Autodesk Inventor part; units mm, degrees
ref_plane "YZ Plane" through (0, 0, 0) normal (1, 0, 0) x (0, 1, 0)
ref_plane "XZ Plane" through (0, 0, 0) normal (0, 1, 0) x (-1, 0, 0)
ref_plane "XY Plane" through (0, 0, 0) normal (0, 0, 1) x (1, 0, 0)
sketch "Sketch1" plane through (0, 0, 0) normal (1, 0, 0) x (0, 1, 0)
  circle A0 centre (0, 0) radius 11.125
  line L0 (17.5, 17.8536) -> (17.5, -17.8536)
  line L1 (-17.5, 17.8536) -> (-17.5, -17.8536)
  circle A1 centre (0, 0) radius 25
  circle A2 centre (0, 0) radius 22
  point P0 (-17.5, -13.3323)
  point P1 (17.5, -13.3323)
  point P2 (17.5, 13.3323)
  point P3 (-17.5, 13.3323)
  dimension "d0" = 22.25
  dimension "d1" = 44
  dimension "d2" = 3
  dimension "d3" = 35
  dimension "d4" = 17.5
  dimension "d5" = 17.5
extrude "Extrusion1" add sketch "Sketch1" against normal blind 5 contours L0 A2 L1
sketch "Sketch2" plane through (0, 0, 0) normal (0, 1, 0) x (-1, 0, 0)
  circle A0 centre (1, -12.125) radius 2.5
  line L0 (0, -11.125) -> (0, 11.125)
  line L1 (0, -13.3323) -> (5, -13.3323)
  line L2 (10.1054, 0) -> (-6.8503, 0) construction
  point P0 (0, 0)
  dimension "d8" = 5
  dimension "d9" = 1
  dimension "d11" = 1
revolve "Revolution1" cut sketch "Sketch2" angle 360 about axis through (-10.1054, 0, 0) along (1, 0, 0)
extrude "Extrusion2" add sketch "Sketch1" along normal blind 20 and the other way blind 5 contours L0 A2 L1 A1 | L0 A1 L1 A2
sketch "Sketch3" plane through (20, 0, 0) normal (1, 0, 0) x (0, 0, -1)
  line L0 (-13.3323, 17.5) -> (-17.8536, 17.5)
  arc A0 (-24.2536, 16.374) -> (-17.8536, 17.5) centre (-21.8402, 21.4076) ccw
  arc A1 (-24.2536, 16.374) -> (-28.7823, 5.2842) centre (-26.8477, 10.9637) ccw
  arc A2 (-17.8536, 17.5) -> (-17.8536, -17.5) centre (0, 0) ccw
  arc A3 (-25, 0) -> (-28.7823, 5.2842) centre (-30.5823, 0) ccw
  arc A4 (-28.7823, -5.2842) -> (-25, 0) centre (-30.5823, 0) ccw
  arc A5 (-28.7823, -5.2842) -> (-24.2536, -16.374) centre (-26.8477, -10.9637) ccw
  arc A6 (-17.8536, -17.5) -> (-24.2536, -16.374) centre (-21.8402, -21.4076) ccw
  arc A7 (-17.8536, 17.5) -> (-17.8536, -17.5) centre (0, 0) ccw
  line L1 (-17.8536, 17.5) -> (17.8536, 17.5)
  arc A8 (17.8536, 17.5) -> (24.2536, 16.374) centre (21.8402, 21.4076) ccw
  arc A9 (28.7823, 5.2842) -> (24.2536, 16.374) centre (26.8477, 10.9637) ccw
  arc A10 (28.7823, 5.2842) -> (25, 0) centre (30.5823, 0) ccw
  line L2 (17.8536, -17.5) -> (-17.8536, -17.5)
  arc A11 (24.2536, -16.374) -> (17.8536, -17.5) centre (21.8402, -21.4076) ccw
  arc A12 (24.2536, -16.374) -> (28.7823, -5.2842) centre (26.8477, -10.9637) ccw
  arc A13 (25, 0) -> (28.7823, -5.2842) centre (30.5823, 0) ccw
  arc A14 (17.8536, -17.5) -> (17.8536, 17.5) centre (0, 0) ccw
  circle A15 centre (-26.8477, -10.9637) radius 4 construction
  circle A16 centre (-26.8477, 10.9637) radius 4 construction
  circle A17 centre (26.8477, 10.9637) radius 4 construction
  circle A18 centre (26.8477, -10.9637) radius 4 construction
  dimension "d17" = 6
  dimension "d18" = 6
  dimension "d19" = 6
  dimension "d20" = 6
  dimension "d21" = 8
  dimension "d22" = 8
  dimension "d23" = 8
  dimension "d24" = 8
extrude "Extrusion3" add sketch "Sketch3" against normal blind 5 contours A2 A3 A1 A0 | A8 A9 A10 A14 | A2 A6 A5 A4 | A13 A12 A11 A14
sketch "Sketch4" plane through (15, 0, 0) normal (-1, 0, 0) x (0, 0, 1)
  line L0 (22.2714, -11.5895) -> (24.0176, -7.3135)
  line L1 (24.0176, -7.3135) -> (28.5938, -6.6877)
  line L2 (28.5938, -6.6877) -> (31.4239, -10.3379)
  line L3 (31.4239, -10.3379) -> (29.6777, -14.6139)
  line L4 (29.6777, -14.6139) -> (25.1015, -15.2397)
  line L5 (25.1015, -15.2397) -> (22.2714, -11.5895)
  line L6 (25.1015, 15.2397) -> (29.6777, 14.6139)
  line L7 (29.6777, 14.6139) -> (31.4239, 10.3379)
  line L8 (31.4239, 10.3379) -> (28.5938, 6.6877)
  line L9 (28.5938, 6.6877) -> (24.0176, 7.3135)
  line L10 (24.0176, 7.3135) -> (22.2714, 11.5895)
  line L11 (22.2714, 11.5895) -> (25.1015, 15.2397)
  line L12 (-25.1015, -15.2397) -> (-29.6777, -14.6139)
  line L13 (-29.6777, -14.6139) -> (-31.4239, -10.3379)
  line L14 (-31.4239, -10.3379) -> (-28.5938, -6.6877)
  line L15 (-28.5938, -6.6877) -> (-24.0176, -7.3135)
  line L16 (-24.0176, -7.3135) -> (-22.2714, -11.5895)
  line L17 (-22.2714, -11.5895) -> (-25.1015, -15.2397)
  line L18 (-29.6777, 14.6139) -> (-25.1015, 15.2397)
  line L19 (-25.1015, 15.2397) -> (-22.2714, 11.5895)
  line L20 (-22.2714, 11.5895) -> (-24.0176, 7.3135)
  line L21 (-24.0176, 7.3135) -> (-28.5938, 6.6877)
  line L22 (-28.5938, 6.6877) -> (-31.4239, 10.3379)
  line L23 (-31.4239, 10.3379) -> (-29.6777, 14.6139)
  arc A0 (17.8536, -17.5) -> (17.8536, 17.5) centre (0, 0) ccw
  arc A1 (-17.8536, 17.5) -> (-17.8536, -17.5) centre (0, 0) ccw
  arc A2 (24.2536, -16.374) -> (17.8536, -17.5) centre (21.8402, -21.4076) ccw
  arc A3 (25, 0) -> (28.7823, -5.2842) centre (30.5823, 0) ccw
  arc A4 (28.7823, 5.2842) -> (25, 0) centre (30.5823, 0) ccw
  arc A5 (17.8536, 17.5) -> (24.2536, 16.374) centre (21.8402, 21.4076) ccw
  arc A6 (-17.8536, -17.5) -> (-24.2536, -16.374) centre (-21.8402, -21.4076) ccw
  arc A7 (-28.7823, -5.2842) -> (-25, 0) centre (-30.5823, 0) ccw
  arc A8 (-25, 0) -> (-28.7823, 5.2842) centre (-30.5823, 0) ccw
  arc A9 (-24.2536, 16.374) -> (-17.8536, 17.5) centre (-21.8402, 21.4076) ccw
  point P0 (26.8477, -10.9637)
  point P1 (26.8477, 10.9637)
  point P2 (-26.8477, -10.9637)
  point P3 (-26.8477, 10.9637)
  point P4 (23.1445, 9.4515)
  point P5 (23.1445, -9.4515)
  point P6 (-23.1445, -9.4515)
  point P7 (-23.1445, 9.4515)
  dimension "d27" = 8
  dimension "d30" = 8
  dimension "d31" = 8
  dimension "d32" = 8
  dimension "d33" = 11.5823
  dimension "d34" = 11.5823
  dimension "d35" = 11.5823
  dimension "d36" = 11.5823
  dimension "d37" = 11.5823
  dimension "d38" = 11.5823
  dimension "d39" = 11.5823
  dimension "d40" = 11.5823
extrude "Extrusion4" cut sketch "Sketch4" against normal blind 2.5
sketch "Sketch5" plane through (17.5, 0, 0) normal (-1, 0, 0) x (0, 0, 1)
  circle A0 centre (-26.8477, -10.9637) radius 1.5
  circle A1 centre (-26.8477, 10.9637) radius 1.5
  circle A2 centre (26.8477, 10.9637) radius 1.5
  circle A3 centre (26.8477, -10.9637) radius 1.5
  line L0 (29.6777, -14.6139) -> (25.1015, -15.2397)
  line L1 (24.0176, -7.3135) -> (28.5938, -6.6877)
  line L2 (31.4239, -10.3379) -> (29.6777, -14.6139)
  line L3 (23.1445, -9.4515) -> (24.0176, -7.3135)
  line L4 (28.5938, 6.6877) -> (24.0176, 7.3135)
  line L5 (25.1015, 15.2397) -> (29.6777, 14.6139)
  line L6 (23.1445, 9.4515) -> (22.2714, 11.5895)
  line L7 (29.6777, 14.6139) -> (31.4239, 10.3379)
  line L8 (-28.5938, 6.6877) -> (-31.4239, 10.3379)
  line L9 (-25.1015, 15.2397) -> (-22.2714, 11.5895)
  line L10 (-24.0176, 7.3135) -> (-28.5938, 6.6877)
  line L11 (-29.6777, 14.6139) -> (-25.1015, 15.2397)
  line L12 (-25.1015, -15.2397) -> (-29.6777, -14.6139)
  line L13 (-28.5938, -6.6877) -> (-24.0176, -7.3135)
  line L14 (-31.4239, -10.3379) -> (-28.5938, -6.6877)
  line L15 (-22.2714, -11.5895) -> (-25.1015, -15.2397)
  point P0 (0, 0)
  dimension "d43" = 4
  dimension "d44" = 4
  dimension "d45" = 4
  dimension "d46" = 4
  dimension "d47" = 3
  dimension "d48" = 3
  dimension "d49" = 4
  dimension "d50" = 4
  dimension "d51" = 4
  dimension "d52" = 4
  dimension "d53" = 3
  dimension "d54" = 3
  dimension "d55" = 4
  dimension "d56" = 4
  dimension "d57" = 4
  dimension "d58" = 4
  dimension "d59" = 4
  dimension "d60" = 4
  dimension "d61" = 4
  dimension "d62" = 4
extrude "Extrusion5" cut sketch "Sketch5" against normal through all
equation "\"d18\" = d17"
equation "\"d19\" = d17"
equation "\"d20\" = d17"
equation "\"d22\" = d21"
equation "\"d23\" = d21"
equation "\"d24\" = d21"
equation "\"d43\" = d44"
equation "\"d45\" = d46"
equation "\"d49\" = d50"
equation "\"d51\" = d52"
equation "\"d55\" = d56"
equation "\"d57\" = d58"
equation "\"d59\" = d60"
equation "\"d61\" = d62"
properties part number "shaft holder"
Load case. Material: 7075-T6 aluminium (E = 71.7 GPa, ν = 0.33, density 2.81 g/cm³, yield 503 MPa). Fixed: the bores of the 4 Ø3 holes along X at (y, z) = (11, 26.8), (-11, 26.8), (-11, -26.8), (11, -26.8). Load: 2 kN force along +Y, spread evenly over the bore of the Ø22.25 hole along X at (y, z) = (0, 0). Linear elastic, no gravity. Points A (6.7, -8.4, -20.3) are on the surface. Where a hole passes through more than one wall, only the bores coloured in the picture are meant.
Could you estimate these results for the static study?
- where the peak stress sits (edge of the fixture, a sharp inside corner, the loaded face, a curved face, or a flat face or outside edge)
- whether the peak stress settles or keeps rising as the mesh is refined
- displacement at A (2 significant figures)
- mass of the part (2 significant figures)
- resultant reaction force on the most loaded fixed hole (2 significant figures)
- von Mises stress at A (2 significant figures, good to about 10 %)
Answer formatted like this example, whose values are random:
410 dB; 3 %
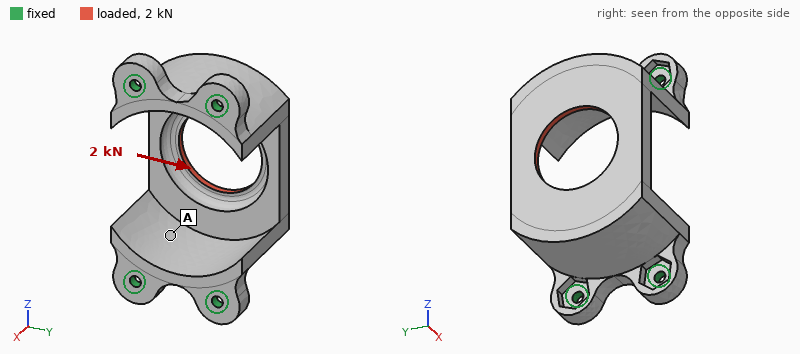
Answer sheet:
edge of the fixture; keeps rising; 32 µm; 32 g; 1.2 kN; 29 MPa
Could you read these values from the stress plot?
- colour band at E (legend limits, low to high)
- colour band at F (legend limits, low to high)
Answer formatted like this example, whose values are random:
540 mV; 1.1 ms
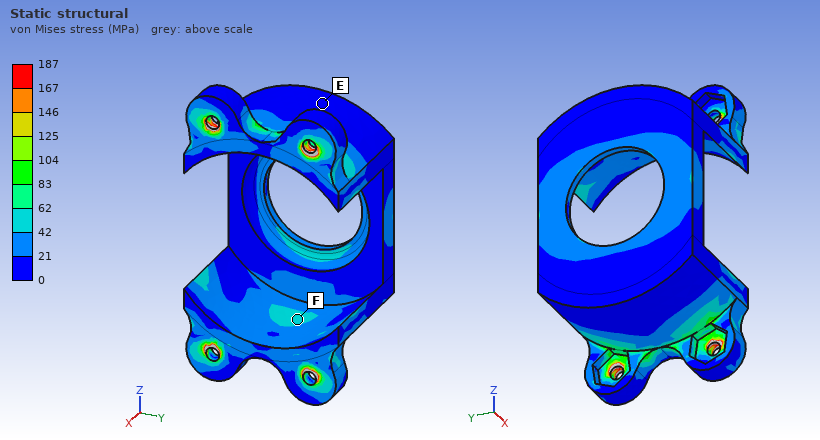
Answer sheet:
0 to 21 MPa; 42 to 62 MPa
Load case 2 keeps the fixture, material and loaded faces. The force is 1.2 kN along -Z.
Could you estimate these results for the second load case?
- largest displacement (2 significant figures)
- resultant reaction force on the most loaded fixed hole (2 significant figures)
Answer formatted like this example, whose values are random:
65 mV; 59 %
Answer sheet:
93 µm; 370 N
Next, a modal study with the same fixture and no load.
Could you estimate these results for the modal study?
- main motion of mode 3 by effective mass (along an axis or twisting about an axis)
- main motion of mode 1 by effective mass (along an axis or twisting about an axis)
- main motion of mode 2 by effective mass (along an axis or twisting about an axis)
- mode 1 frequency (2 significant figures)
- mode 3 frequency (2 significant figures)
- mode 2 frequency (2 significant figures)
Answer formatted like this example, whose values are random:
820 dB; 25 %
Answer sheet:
twisting about X; along Z; along Y; 4300 Hz; 7500 Hz; 6600 Hz
